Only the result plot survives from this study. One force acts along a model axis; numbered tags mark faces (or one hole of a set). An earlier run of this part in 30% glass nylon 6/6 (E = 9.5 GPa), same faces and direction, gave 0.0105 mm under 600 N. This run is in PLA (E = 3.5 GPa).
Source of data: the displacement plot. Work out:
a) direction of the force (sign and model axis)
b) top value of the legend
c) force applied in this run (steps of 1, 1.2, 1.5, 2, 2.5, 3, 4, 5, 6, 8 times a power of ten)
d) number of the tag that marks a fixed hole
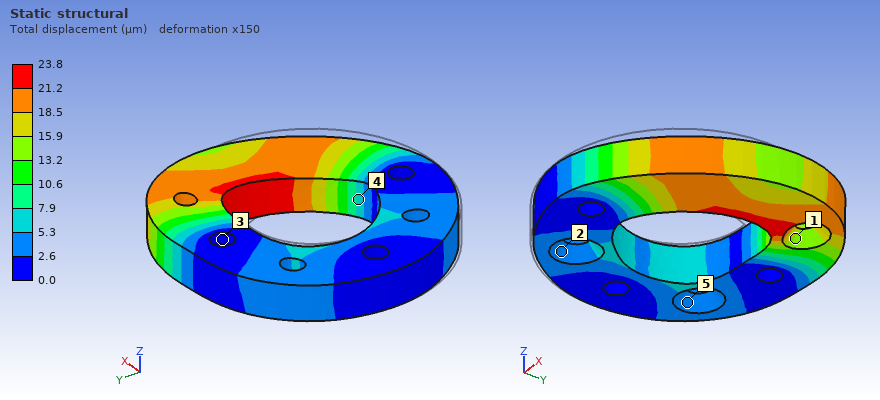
+Y
23.8 µm
500 N
3
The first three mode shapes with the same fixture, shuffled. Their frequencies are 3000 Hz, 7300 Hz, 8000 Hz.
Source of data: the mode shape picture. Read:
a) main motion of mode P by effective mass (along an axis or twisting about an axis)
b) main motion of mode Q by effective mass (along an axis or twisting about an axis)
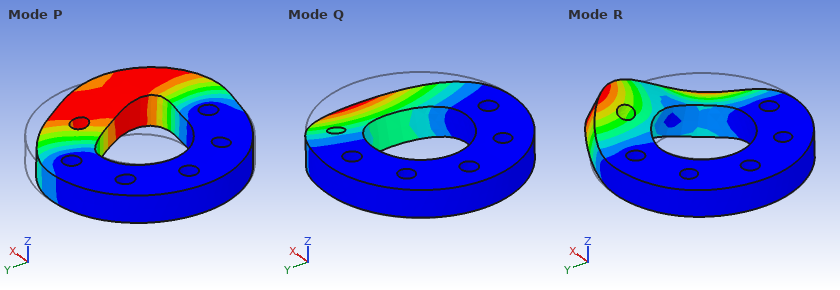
along Y
along Z
